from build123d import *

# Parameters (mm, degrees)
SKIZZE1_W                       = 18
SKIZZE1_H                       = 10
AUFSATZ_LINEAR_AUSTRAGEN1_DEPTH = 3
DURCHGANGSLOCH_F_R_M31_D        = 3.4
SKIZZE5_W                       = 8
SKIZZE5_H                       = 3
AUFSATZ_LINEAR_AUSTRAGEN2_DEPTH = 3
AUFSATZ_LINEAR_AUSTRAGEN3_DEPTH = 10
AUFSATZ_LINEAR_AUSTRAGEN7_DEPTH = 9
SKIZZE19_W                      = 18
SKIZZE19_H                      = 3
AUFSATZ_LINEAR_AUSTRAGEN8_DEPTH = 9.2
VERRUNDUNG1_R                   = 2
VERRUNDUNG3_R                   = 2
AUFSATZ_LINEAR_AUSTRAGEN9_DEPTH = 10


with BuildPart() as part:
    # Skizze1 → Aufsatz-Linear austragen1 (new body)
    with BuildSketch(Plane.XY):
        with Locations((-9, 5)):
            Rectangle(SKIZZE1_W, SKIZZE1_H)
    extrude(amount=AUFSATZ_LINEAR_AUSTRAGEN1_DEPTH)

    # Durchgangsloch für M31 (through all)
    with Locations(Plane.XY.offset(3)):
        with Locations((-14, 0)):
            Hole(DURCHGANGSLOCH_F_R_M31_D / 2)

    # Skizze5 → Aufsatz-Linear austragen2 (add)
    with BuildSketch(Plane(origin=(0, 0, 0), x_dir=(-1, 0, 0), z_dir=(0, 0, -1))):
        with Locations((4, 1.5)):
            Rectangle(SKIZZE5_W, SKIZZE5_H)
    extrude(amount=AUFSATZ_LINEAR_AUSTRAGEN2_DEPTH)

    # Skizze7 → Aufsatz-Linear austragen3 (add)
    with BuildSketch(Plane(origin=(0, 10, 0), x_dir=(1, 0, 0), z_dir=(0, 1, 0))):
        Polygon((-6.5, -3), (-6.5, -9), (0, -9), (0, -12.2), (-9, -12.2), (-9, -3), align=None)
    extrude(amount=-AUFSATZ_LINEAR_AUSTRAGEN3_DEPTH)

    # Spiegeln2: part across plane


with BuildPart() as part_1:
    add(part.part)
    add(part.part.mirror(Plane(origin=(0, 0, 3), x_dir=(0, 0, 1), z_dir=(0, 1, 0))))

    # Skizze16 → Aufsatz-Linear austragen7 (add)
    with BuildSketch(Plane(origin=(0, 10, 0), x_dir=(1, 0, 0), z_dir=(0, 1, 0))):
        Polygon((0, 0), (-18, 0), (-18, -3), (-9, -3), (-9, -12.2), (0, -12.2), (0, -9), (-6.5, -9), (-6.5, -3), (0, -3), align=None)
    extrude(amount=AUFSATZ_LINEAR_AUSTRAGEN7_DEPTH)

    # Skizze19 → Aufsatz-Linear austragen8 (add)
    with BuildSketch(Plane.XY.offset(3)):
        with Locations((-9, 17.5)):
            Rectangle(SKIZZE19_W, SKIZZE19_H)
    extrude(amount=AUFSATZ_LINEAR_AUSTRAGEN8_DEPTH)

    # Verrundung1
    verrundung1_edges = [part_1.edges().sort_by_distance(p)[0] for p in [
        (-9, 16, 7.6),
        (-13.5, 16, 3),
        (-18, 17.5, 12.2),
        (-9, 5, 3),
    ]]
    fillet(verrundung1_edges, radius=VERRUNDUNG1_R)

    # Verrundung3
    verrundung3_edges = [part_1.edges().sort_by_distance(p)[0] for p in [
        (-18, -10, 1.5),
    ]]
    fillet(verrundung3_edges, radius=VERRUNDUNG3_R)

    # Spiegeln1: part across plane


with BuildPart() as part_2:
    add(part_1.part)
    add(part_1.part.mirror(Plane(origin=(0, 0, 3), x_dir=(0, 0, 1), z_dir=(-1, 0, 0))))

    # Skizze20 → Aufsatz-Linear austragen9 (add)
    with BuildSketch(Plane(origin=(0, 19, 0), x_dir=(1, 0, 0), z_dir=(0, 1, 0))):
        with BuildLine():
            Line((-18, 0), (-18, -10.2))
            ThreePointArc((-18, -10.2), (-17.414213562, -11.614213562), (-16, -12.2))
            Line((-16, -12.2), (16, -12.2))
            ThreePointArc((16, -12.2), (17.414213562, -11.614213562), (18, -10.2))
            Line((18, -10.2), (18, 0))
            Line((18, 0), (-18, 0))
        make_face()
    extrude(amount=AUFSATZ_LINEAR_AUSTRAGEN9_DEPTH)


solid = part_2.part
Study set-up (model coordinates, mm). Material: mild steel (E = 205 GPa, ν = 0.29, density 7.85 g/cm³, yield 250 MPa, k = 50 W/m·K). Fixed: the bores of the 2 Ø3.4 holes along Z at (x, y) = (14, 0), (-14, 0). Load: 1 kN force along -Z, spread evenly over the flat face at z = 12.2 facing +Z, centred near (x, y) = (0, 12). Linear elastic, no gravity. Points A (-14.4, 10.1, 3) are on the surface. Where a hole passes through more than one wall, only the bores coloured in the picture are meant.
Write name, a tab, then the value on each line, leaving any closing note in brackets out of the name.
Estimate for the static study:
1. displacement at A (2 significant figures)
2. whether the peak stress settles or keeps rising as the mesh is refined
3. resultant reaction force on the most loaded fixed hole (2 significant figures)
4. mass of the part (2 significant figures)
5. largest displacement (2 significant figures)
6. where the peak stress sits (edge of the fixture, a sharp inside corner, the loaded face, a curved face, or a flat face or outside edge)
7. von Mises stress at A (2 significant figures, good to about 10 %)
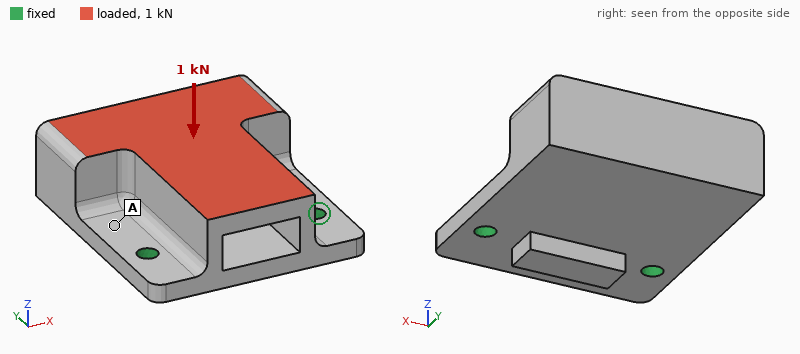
displacement at A	20 µm
whether the peak stress settles or keeps rising as the mesh is refined	keeps rising
resultant reaction force on the most loaded fixed hole	520 N
mass of the part	87 g
largest displacement	67 µm
where the peak stress sits	edge of the fixture
von Mises stress at A	26 MPa
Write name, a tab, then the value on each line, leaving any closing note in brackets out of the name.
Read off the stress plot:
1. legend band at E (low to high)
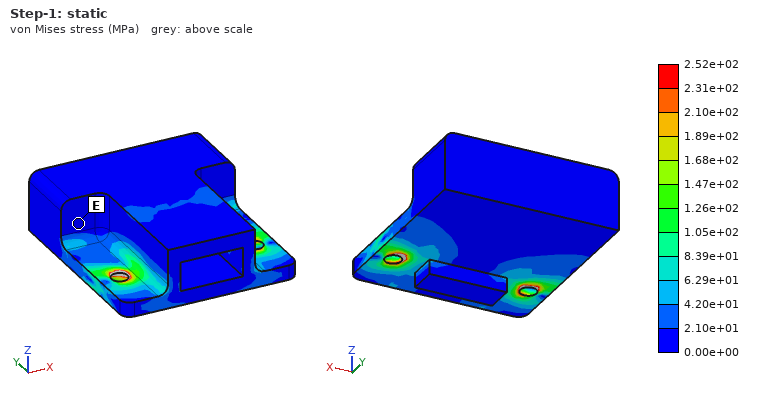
legend band at E	0.00e+00 to 2.10e+01 MPa
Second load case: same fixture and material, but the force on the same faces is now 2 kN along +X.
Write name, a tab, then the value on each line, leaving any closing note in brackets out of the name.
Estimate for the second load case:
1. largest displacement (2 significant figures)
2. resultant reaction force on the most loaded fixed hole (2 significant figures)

largest displacement	17 µm
resultant reaction force on the most loaded fixed hole	1.6 kN
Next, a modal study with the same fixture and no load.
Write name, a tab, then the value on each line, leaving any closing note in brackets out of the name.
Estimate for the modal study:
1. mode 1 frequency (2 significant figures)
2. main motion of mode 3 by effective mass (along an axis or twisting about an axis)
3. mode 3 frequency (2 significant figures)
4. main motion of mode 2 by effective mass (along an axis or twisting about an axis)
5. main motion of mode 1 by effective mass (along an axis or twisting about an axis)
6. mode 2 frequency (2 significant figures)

mode 1 frequency	2300 Hz
main motion of mode 3 by effective mass	along X
mode 3 frequency	11 kHz
main motion of mode 2 by effective mass	along X
main motion of mode 1 by effective mass	along Z
mode 2 frequency	8600 Hz
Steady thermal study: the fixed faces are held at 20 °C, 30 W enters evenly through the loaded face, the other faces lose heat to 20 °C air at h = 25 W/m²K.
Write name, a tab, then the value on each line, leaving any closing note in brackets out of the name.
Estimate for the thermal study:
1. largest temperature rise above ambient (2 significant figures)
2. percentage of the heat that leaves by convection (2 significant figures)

largest temperature rise above ambient	61 K
percentage of the heat that leaves by convection	16 %
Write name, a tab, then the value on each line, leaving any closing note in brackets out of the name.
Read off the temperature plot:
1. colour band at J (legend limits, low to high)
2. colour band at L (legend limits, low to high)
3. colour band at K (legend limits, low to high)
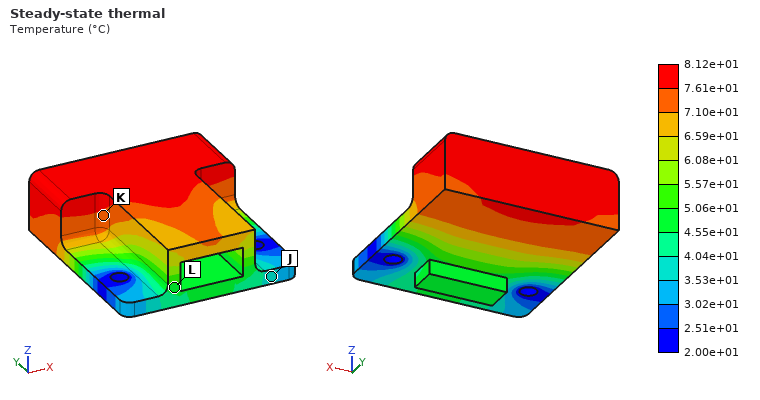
colour band at J	3.53e+01 to 4.04e+01 °C
colour band at L	4.55e+01 to 5.06e+01 °C
colour band at K	7.10e+01 to 7.61e+01 °C
